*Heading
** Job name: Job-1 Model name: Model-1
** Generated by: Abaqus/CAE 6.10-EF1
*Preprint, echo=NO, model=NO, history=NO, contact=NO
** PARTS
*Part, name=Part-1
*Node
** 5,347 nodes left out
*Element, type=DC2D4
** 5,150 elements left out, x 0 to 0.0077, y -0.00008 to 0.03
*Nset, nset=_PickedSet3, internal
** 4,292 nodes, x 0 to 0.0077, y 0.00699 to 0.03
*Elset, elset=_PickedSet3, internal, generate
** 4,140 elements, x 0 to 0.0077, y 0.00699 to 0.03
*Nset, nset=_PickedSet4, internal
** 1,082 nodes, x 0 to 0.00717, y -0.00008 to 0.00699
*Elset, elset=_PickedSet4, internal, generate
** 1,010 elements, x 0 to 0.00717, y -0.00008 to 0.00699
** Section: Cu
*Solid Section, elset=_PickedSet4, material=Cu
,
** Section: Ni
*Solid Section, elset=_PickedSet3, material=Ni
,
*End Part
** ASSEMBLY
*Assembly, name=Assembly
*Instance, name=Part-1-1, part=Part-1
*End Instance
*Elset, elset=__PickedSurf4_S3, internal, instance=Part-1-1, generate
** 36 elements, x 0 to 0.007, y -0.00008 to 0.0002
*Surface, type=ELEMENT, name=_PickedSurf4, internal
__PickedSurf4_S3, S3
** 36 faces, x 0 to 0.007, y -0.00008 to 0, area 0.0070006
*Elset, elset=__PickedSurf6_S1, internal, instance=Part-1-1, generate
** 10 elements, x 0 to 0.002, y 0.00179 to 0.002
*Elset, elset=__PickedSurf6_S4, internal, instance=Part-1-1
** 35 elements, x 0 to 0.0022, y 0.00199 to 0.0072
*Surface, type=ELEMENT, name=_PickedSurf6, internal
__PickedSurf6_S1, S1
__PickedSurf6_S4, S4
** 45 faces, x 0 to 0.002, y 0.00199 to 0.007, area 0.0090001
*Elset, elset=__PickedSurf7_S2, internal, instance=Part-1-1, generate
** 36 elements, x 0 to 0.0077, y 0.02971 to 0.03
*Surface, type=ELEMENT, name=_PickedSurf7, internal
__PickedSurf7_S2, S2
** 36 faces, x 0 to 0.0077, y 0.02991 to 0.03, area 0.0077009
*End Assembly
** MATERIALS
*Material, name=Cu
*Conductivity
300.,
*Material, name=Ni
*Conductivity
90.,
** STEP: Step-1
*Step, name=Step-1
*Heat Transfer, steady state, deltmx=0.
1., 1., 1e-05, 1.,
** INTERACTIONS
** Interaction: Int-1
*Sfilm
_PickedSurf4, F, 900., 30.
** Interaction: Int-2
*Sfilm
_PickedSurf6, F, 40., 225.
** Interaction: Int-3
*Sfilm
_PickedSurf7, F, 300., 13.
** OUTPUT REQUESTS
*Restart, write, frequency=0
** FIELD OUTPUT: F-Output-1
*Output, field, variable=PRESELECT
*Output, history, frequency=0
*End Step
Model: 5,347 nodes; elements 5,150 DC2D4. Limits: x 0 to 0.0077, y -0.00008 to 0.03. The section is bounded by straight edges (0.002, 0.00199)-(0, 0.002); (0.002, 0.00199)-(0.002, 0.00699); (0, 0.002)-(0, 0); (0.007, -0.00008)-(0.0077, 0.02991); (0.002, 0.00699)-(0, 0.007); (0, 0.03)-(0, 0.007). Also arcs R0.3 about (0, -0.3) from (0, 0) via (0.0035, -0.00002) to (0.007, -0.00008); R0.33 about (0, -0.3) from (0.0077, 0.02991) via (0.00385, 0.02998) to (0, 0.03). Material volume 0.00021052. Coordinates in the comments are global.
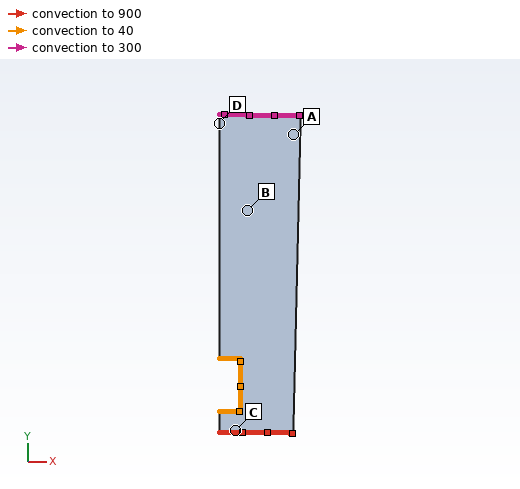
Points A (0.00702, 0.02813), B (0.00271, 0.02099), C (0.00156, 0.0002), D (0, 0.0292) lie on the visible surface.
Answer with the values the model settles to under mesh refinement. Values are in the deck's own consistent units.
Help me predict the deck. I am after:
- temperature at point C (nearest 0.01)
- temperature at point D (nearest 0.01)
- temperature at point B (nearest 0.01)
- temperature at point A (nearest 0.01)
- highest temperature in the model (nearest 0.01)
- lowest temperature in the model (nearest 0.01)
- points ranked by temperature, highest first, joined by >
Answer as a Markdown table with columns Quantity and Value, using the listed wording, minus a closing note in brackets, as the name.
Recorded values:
| Quantity | Value |
|---|---|
| temperature at point C | 128.84 |
| temperature at point D | 128.94 |
| temperature at point B | 128.73 |
| temperature at point A | 128.91 |
| highest temperature in the model | 128.96 |
| lowest temperature in the model | 128.01 |
| points ranked by temperature, highest first, joined by > | D > A > C > B |
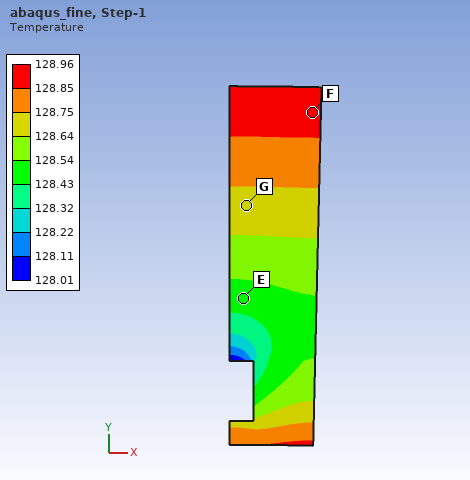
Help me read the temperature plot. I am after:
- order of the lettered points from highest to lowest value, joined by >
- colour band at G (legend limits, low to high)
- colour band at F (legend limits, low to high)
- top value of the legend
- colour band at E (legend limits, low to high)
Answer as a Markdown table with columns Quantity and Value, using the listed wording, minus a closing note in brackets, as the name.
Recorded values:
| Quantity | Value |
|---|---|
| order of the lettered points from highest to lowest value, joined by > | F > G > E |
| colour band at G | 128.64 to 128.75 |
| colour band at F | 128.85 to 128.96 |
| top value of the legend | 128.96 |
| colour band at E | 128.43 to 128.54 |
